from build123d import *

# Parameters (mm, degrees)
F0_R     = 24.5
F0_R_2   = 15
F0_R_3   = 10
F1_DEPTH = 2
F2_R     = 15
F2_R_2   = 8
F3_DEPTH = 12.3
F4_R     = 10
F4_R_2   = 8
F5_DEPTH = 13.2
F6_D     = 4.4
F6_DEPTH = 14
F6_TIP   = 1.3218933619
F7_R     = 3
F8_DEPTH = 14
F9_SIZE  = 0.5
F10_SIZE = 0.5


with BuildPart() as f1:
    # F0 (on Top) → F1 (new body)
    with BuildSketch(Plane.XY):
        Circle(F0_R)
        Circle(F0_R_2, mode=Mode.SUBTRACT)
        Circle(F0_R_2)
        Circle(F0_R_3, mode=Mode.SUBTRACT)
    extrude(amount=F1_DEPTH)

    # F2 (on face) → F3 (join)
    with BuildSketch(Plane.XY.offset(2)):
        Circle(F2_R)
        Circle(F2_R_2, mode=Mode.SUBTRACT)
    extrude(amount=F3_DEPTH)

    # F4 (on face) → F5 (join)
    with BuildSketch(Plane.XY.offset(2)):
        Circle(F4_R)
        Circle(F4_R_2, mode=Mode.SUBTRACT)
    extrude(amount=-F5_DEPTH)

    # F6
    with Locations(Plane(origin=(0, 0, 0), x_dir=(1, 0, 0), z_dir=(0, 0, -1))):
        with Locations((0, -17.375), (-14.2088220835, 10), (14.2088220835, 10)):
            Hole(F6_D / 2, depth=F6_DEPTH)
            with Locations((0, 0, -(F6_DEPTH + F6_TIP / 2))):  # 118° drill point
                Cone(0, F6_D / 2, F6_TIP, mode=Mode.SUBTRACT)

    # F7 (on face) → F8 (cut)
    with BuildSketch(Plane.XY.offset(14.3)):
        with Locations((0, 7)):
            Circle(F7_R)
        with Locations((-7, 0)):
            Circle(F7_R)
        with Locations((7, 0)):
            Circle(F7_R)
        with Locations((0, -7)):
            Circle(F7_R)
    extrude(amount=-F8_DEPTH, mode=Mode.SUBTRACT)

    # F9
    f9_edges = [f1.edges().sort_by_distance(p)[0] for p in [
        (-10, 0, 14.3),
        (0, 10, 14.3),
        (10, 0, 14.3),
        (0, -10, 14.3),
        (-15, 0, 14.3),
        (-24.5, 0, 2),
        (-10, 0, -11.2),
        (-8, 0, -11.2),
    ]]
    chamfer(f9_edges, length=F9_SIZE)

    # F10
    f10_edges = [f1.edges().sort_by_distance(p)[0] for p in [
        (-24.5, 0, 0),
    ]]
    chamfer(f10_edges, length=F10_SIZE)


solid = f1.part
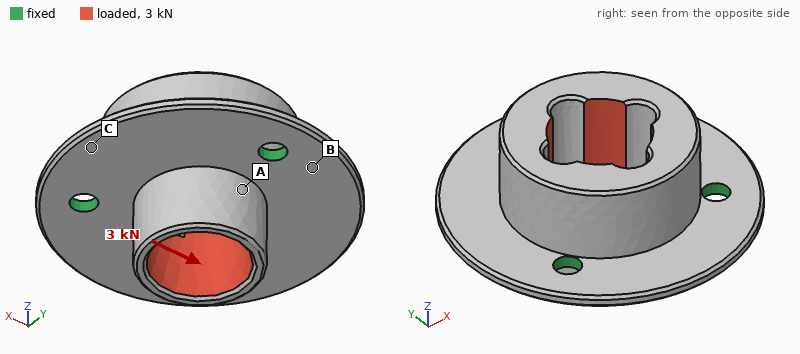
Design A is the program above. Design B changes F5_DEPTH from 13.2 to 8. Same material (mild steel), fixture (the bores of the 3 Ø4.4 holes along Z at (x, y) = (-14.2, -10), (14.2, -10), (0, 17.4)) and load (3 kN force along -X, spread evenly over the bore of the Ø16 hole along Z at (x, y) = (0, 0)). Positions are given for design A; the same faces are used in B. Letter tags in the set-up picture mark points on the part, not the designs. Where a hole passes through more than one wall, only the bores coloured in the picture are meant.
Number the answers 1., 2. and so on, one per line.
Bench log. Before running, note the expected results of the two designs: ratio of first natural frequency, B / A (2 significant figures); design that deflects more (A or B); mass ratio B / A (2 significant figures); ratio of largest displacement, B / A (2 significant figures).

1. 1.0
2. A
3. 0.94
4. 0.52
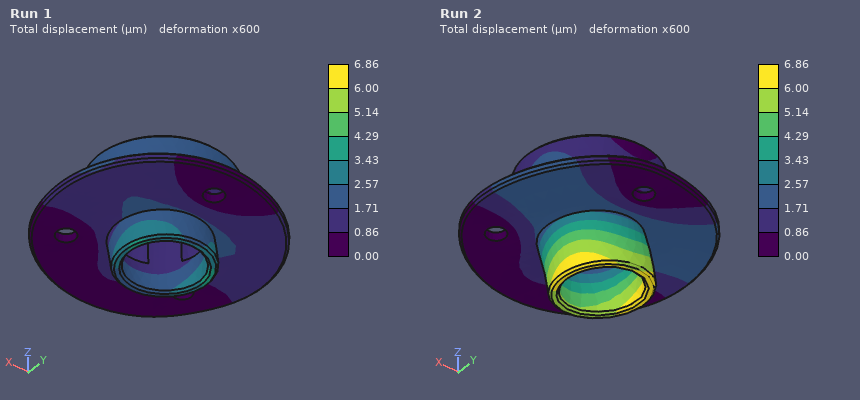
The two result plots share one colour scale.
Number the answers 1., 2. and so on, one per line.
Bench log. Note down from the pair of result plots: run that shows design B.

1. Run 1
